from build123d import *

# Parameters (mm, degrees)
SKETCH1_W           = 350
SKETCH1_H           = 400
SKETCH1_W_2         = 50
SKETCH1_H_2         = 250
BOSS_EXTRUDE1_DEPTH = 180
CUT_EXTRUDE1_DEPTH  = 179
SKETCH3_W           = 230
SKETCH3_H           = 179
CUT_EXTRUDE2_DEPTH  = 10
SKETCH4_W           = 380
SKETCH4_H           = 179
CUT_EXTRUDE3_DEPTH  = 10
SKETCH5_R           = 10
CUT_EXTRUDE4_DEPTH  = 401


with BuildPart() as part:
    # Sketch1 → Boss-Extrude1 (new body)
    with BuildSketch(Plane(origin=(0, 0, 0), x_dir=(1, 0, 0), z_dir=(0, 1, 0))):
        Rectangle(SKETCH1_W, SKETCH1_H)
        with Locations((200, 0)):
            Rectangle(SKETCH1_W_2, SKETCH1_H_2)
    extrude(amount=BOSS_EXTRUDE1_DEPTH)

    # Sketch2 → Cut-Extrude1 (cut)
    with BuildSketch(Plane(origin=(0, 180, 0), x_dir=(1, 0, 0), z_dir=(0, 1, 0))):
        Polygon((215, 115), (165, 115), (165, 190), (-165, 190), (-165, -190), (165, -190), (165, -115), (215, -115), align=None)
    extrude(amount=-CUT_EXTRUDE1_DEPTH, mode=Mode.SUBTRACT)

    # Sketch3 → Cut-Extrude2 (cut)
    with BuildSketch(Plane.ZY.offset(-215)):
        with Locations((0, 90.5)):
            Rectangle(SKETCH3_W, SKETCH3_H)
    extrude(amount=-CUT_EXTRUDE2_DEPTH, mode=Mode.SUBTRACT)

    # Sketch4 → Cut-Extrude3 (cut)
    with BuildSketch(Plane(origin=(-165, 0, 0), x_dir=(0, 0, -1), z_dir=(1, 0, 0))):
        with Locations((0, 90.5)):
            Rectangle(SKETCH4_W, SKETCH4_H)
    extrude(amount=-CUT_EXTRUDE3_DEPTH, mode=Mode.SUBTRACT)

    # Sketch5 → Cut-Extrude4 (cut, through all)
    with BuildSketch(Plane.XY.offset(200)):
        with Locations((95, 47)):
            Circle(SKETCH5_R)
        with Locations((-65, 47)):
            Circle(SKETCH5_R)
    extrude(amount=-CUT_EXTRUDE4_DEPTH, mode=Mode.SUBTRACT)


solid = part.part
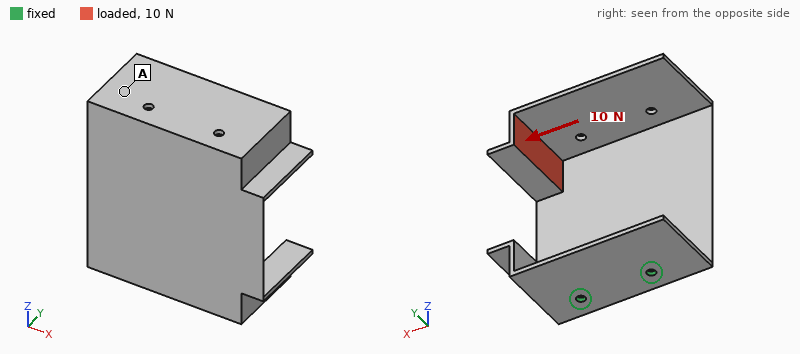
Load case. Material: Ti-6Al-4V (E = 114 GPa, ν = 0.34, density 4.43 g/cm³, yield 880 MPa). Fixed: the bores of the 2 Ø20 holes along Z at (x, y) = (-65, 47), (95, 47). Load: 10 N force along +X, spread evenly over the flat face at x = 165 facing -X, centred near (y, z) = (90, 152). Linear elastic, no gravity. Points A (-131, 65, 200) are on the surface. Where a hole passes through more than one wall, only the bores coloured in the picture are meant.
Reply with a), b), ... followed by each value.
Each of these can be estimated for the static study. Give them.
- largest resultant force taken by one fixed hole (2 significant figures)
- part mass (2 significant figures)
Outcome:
a) 20 N
b) 8.2 kg
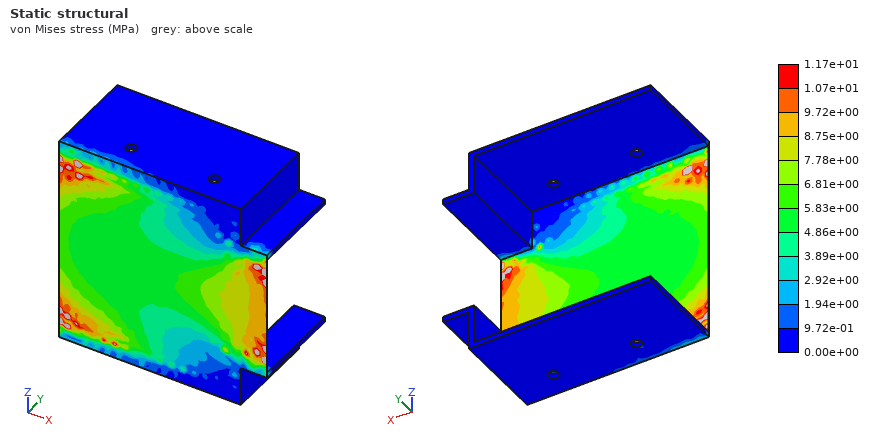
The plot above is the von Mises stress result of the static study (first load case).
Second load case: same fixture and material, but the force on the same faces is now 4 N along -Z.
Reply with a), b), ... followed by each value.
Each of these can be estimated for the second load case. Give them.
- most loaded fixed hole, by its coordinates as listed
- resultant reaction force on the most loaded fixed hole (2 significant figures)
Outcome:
a) (95, 47)
b) 4.8 N
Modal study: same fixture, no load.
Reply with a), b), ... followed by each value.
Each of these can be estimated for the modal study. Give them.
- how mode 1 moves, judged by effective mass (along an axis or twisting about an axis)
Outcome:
a) along Y
